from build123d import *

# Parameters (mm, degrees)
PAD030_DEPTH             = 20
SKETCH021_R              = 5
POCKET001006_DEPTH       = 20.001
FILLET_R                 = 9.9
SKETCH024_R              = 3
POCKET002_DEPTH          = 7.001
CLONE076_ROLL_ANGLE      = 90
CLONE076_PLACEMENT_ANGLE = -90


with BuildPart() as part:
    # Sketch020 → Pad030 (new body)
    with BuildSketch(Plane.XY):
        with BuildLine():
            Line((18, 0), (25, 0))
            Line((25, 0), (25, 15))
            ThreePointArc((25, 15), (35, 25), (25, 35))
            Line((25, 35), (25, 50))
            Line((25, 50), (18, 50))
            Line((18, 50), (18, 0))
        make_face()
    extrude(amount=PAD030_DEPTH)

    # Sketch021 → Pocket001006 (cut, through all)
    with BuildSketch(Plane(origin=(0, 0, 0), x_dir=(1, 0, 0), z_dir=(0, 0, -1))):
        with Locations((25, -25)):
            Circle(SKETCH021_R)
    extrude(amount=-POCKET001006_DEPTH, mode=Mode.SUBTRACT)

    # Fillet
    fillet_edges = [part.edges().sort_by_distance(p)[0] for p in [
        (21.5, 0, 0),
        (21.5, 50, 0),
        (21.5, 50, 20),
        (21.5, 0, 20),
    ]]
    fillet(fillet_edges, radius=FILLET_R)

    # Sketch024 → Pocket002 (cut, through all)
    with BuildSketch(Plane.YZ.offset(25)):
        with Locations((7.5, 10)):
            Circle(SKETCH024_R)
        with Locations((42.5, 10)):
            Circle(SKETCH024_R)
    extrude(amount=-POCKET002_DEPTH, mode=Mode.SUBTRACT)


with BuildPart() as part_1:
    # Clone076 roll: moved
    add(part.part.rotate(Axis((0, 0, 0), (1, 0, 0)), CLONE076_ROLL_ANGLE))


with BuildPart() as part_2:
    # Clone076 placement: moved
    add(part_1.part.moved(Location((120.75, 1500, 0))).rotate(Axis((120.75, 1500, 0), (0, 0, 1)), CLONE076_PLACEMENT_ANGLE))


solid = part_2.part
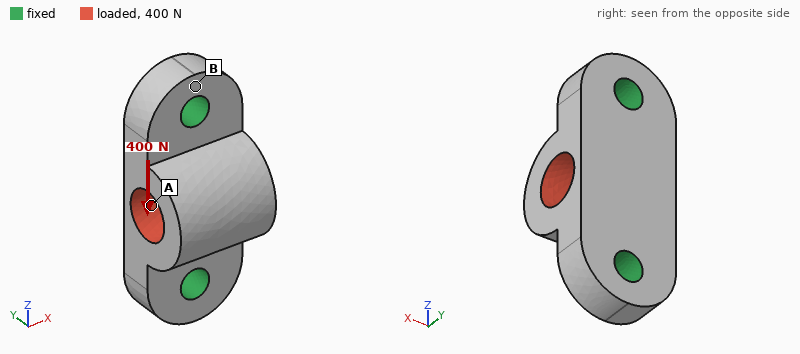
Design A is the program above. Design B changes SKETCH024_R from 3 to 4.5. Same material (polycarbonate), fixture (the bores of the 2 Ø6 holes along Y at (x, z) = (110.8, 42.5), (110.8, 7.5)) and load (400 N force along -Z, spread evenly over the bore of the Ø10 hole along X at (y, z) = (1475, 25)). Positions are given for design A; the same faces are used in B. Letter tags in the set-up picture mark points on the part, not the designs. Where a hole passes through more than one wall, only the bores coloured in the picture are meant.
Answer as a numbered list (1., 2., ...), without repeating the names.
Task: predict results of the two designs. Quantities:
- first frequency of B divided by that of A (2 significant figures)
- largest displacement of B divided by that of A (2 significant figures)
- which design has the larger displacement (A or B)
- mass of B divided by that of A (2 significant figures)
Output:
1. 1.2
2. 0.88
3. A
4. 0.93
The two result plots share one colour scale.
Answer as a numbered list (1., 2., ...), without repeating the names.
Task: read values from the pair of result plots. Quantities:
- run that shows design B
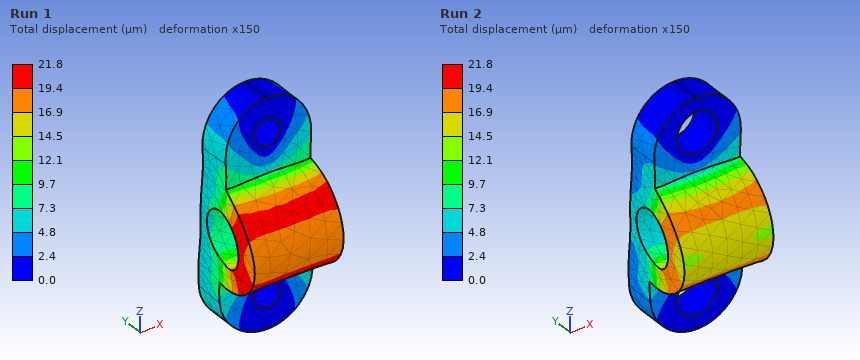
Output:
1. Run 2
